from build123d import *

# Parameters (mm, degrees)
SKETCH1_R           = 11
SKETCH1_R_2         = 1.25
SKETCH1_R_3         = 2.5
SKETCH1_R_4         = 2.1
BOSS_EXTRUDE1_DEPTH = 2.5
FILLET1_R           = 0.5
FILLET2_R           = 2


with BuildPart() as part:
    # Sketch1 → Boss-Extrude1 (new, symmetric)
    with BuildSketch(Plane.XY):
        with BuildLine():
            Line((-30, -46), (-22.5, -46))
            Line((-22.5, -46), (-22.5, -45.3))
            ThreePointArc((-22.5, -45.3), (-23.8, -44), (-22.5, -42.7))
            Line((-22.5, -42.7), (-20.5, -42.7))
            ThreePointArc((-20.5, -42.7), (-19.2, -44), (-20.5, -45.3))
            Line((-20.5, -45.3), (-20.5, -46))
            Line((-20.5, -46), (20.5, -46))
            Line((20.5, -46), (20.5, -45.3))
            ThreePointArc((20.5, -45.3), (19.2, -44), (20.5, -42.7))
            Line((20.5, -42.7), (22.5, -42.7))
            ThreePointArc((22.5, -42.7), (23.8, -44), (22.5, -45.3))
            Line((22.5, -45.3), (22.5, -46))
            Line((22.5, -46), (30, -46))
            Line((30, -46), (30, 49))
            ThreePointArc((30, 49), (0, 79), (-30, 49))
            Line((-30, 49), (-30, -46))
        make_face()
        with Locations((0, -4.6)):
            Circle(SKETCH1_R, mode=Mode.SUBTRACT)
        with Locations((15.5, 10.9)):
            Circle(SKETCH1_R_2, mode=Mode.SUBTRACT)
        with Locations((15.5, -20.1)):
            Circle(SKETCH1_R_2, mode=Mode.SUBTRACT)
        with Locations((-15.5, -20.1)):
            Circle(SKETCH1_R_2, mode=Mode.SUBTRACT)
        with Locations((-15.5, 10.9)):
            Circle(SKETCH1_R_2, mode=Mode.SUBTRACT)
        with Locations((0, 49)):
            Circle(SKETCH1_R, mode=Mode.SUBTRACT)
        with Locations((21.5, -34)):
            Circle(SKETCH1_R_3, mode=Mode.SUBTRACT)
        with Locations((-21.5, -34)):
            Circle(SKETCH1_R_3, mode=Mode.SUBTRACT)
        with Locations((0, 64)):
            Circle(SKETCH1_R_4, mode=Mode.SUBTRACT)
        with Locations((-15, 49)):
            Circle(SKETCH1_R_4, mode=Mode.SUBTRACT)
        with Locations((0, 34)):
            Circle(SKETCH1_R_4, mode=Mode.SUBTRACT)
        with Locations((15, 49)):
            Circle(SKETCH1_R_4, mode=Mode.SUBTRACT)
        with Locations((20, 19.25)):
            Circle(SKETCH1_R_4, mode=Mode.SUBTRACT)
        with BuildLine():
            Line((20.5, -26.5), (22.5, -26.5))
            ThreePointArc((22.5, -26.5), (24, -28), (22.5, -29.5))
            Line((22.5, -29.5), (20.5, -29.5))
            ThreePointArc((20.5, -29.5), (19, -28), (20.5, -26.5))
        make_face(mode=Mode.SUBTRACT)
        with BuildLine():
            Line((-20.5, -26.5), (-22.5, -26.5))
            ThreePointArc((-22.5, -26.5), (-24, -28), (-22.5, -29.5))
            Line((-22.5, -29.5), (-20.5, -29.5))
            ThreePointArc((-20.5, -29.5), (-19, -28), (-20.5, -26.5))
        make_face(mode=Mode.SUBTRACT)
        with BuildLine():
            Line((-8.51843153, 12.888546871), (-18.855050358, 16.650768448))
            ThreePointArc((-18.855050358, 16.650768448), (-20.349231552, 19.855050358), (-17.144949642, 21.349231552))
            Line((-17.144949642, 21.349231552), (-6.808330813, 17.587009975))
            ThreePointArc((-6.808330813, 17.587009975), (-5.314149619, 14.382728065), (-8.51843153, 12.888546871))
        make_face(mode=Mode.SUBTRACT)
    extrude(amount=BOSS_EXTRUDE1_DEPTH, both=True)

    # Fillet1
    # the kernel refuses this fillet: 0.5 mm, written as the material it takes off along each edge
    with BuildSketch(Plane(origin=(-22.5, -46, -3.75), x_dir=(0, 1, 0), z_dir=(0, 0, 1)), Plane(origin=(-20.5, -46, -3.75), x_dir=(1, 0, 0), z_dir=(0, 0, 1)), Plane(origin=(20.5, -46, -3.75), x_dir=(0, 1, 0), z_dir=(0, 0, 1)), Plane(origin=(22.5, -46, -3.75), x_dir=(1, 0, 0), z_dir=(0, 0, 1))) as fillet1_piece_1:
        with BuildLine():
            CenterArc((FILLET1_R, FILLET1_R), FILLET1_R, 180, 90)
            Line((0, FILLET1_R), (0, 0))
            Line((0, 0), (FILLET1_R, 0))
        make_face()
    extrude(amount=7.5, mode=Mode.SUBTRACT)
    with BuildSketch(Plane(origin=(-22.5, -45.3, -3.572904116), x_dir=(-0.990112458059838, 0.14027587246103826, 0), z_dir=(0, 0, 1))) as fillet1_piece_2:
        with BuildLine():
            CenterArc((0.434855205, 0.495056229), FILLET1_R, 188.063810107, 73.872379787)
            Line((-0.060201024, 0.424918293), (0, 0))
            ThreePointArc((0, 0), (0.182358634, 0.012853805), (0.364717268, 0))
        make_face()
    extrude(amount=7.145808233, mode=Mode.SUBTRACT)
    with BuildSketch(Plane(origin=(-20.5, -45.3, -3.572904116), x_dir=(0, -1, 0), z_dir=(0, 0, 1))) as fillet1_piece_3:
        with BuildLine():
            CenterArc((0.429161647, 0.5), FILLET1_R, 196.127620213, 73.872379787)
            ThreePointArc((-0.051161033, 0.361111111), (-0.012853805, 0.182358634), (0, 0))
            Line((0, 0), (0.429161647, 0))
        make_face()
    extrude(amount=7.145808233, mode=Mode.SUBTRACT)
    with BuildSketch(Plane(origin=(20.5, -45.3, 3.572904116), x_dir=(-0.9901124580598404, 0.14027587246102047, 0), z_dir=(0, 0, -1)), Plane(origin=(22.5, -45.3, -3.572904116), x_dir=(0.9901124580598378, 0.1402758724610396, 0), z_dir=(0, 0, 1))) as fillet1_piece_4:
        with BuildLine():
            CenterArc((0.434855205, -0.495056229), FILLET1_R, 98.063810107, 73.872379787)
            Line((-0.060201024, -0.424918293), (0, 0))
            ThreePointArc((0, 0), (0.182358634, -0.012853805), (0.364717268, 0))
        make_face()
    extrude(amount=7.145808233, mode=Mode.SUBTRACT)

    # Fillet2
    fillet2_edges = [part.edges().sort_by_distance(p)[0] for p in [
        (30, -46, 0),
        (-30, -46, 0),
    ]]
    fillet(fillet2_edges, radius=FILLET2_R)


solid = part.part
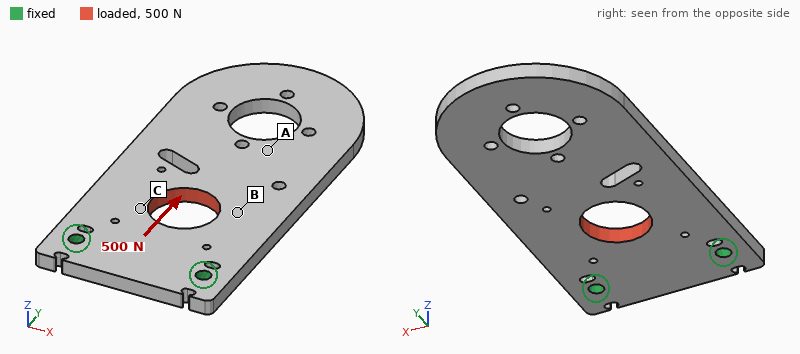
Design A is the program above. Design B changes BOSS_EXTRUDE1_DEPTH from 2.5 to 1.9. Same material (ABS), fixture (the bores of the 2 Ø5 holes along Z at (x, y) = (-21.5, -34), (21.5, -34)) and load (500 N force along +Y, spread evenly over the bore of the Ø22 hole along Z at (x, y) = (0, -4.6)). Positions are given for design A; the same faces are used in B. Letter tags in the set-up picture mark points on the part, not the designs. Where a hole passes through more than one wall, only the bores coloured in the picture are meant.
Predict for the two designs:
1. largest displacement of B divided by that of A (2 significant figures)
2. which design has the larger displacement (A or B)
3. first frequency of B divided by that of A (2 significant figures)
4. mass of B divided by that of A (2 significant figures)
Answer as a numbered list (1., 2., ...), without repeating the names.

1. 1.3
2. B
3. 0.77
4. 0.76
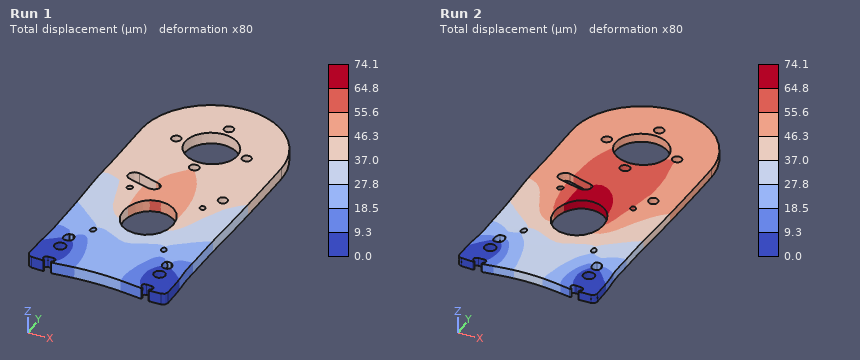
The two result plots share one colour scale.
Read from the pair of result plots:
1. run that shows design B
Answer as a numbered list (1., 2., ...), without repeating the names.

1. Run 2
